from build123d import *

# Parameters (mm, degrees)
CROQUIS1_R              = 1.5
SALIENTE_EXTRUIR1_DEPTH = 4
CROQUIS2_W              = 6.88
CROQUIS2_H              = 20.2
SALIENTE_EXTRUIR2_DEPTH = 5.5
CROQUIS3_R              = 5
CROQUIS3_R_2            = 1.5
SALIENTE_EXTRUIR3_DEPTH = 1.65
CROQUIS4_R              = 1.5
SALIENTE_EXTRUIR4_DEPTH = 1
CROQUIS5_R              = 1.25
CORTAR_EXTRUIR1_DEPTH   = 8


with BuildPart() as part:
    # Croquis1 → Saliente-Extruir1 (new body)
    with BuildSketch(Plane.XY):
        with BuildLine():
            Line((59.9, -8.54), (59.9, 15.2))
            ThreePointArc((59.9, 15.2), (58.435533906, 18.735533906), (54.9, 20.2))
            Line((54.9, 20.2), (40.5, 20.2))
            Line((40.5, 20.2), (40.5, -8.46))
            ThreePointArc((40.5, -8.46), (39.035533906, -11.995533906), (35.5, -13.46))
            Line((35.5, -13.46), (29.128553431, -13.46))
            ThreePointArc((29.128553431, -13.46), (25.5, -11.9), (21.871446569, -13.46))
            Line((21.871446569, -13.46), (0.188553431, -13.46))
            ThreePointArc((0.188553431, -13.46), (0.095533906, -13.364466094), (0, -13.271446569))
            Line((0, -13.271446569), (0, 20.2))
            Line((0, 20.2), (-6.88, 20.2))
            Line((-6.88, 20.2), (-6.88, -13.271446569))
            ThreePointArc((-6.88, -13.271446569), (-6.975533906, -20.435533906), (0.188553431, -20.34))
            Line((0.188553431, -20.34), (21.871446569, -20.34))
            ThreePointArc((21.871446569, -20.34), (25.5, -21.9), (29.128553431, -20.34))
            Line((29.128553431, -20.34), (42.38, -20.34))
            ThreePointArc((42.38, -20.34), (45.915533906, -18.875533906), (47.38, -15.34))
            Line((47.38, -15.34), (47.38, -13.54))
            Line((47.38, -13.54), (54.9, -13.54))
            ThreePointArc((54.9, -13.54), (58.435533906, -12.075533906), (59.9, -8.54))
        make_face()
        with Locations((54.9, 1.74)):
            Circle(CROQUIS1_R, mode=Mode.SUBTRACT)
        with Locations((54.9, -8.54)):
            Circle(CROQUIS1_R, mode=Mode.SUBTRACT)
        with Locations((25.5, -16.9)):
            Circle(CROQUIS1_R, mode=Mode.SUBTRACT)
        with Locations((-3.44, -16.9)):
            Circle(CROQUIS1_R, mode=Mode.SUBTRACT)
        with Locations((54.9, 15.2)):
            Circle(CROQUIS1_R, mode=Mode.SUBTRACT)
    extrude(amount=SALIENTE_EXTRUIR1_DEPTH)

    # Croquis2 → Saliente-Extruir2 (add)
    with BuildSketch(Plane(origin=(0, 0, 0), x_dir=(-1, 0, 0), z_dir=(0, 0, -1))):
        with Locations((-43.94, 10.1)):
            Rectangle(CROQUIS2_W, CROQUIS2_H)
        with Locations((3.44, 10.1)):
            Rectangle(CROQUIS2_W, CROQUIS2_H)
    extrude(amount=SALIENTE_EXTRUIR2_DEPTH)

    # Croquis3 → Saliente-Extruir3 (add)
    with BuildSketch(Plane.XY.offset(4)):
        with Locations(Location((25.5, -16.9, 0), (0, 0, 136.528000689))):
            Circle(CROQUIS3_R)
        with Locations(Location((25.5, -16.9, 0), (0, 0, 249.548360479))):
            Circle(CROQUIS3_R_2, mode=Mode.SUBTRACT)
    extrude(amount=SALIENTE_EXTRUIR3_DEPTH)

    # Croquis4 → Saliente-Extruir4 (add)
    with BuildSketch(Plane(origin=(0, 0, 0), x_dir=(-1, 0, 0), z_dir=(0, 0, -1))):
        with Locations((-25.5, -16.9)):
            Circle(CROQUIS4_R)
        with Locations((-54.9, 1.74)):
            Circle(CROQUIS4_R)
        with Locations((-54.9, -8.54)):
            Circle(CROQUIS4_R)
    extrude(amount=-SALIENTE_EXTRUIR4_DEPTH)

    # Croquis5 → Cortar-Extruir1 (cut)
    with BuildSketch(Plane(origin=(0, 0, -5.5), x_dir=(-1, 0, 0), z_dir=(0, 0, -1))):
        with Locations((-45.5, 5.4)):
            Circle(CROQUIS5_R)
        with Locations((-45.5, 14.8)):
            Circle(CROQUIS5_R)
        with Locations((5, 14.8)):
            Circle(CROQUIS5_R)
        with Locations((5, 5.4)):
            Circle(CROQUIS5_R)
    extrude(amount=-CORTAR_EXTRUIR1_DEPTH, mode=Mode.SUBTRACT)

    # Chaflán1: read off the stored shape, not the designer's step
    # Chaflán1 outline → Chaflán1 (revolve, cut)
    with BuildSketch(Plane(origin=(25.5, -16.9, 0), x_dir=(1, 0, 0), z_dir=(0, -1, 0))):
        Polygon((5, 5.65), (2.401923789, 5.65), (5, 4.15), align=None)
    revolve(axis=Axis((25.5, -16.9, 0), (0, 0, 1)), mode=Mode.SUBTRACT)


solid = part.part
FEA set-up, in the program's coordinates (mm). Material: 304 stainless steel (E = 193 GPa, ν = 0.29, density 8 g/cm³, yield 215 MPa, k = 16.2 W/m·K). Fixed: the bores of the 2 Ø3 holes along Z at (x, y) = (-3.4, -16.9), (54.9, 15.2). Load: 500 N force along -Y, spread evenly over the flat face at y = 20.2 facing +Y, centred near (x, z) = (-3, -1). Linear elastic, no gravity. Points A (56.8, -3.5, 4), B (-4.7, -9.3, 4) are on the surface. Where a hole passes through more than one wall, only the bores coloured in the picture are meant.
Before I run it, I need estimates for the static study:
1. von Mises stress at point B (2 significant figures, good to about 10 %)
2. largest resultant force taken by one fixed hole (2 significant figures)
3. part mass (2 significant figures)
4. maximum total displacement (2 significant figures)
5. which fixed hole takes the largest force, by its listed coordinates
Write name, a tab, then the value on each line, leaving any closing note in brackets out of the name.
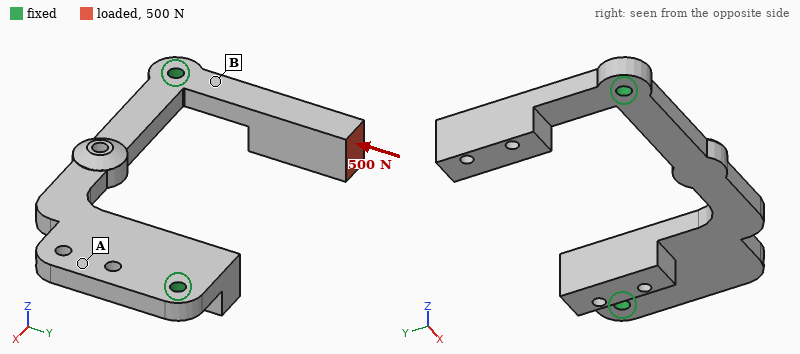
von Mises stress at point B	56 MPa
largest resultant force taken by one fixed hole	500 N
part mass	51 g
maximum total displacement	97 µm
which fixed hole takes the largest force, by its listed coordinates	(-3.4, -16.9)
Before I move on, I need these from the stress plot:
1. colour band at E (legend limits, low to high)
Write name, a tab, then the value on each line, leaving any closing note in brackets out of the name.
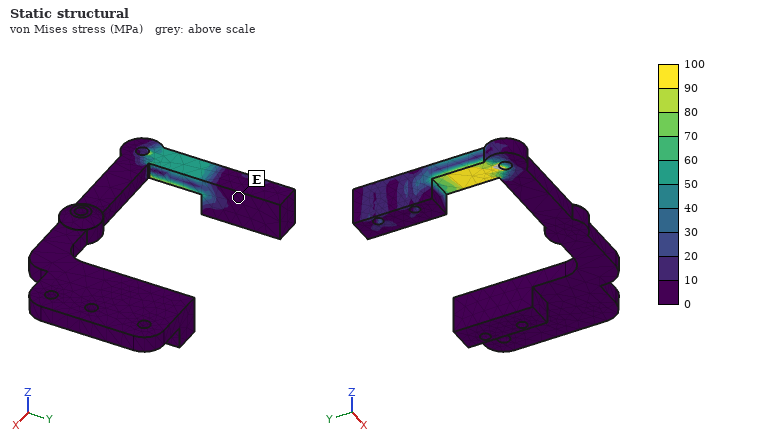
colour band at E	0 to 10 MPa
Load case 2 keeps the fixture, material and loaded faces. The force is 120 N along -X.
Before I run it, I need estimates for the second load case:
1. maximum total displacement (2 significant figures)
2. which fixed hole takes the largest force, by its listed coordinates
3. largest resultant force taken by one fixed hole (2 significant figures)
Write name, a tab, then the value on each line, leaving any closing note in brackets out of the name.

maximum total displacement	0.10 mm
which fixed hole takes the largest force, by its listed coordinates	(-3.4, -16.9)
largest resultant force taken by one fixed hole	140 N
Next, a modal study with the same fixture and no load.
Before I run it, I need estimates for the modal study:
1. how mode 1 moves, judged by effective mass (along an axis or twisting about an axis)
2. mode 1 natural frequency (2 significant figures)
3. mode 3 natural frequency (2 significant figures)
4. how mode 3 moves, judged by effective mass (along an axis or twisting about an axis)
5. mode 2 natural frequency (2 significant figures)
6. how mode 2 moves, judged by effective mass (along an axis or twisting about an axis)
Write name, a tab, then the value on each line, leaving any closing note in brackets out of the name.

how mode 1 moves, judged by effective mass	along Z
mode 1 natural frequency	1700 Hz
mode 3 natural frequency	3000 Hz
how mode 3 moves, judged by effective mass	along Z
mode 2 natural frequency	2600 Hz
how mode 2 moves, judged by effective mass	along X
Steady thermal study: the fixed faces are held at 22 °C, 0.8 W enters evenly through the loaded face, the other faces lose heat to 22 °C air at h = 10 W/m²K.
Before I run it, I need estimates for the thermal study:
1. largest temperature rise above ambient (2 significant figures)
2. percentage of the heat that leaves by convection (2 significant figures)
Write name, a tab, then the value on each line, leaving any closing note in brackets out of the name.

largest temperature rise above ambient	36 K
percentage of the heat that leaves by convection	34 %
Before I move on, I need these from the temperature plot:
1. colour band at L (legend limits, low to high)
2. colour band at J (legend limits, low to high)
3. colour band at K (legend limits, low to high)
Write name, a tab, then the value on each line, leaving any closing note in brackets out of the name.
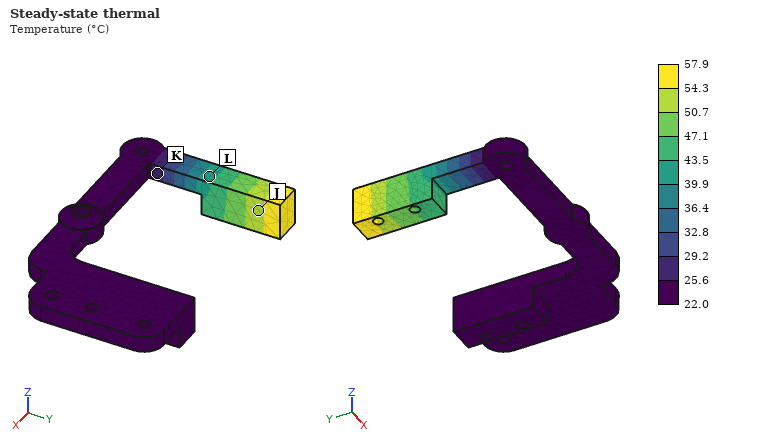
colour band at L	39.9 to 43.5 °C
colour band at J	50.7 to 54.3 °C
colour band at K	25.6 to 29.2 °C
